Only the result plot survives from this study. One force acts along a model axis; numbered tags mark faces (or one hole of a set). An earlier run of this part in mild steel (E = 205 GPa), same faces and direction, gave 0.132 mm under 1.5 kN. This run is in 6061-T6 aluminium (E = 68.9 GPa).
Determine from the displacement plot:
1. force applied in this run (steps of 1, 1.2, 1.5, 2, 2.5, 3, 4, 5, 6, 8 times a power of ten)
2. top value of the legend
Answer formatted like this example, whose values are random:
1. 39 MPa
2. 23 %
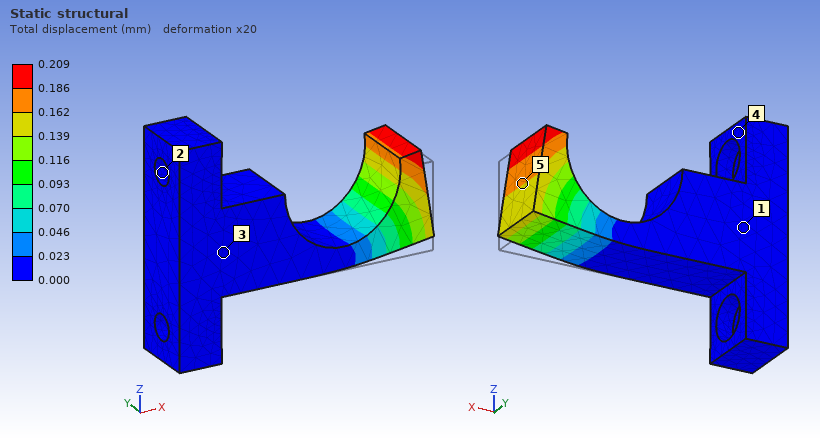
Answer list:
1. 800 N
2. 0.209 mm
